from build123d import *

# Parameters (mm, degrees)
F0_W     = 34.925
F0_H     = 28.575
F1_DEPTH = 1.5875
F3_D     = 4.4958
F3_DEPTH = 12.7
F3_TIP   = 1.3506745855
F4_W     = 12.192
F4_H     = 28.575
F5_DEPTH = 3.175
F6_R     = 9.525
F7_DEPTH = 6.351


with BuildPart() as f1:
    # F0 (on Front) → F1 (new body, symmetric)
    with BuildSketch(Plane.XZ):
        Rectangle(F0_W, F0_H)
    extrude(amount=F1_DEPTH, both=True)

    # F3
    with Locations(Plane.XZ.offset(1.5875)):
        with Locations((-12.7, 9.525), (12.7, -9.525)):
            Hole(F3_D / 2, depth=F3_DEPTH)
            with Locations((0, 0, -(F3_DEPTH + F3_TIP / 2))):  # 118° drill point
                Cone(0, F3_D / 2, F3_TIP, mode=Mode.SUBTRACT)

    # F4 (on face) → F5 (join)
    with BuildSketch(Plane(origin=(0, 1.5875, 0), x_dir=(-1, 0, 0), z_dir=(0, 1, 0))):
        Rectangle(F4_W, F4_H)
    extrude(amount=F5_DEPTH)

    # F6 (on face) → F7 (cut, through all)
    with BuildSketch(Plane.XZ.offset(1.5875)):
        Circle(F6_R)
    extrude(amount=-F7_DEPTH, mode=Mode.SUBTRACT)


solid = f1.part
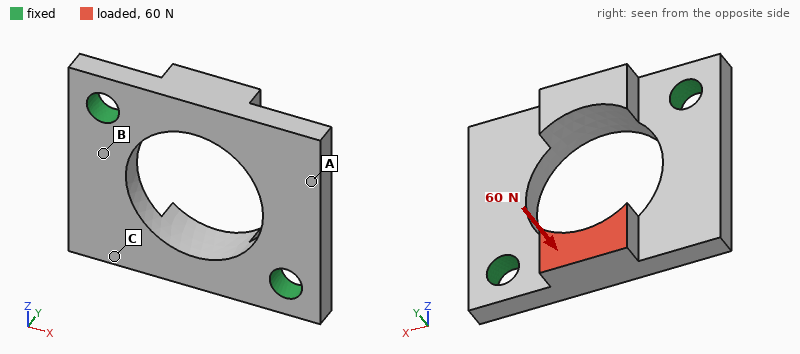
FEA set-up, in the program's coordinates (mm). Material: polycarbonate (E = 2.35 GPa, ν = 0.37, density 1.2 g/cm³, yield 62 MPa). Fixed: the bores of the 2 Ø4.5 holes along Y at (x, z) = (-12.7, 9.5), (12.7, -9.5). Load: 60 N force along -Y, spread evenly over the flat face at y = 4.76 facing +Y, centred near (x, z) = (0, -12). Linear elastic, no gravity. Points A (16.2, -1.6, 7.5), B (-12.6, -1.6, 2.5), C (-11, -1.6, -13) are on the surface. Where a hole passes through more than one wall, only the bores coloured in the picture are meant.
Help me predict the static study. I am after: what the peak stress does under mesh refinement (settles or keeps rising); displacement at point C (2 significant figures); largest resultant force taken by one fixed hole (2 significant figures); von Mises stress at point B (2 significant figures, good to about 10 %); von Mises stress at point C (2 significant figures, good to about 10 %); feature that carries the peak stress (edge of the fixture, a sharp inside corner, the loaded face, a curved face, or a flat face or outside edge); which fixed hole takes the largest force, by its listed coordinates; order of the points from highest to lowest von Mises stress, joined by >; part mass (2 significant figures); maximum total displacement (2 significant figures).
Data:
keeps rising
0.40 mm
46 N
8.5 MPa
4.3 MPa
edge of the fixture
(12.7, -9.5)
B > C > A
3.1 g
0.47 mm
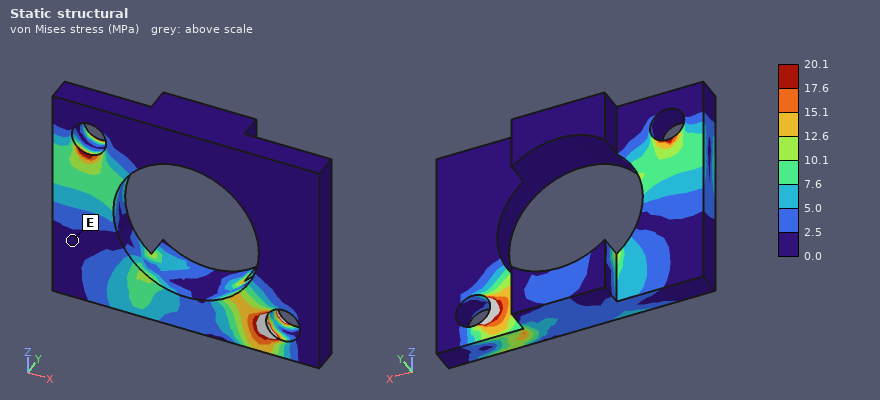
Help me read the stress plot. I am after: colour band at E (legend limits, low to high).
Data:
0.0 to 2.5 MPa
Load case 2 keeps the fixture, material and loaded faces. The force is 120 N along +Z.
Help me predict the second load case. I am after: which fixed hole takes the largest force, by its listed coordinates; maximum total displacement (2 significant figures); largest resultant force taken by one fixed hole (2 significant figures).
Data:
(12.7, -9.5)
0.44 mm
72 N
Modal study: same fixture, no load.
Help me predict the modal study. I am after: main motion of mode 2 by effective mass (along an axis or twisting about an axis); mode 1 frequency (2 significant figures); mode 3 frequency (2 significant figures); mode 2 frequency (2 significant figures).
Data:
along Y
1800 Hz
5900 Hz
1900 Hz
